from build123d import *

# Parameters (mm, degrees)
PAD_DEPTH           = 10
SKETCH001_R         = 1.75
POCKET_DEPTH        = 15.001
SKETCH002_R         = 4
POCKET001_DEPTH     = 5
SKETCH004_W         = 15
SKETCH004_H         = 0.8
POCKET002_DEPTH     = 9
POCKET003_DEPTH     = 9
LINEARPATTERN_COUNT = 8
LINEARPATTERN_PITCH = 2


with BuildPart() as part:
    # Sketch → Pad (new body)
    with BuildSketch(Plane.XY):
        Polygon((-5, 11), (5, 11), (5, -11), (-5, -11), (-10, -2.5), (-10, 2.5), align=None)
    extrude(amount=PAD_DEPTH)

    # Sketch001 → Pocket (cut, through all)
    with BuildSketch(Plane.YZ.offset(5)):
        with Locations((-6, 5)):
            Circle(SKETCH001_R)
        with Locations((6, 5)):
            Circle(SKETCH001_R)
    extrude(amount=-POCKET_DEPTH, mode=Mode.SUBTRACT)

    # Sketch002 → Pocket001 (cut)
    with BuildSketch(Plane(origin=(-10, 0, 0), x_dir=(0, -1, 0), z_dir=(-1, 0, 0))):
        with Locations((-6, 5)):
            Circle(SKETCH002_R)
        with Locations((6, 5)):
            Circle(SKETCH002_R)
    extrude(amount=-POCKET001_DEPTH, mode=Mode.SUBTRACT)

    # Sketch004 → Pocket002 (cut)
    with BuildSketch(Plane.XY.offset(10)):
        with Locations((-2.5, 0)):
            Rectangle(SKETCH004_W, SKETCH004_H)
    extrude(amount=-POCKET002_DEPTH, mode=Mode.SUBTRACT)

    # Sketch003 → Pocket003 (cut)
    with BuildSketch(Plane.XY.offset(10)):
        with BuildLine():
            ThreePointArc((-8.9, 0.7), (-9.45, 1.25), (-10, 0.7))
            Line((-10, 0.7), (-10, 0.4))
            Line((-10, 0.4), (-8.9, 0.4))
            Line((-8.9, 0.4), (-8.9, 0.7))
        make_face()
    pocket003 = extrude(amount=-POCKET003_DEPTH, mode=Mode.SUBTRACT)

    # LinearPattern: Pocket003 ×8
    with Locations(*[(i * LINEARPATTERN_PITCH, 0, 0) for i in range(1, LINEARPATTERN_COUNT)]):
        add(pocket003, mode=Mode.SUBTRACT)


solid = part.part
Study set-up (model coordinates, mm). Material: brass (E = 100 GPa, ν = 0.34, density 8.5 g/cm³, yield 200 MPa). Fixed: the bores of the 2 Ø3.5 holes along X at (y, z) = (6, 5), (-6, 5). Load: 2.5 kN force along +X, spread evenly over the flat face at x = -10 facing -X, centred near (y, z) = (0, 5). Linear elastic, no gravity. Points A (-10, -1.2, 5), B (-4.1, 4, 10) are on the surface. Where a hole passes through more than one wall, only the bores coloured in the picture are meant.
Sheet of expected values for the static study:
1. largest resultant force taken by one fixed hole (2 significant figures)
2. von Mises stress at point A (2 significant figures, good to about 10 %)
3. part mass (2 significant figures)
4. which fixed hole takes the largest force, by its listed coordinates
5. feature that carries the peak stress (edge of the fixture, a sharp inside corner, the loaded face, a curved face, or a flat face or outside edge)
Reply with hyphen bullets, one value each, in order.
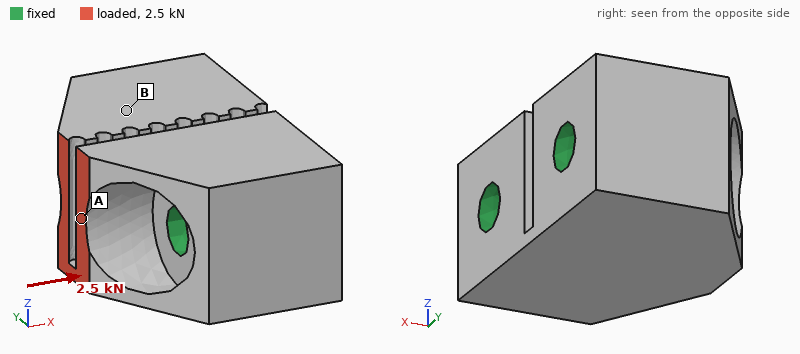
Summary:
- 1.3 kN
- 64 MPa
- 19 g
- (-6, 5)
- the loaded face
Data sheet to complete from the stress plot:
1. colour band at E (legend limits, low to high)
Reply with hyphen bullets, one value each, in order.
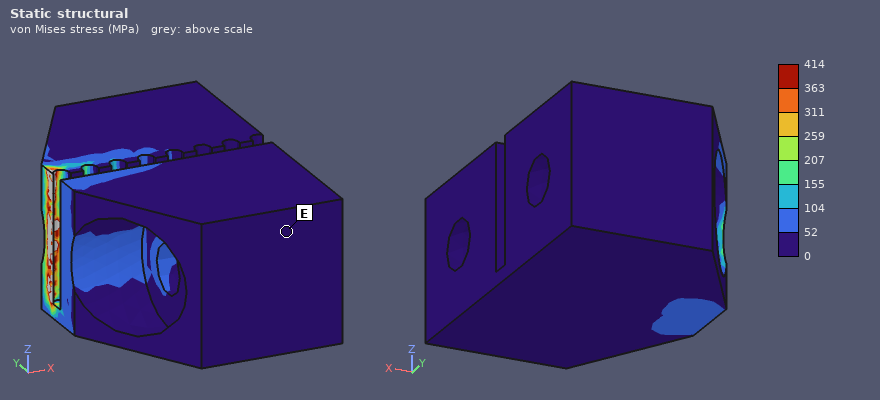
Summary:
- 0 to 52 MPa
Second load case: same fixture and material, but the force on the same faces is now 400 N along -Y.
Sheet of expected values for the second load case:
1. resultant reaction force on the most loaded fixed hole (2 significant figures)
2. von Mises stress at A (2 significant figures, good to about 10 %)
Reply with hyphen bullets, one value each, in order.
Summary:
- 230 N
- 29 MPa
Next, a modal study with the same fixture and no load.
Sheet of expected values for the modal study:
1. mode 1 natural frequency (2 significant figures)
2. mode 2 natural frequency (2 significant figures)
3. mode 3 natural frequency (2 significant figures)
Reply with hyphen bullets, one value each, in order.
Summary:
- 41 kHz
- 44 kHz
- 48 kHz
